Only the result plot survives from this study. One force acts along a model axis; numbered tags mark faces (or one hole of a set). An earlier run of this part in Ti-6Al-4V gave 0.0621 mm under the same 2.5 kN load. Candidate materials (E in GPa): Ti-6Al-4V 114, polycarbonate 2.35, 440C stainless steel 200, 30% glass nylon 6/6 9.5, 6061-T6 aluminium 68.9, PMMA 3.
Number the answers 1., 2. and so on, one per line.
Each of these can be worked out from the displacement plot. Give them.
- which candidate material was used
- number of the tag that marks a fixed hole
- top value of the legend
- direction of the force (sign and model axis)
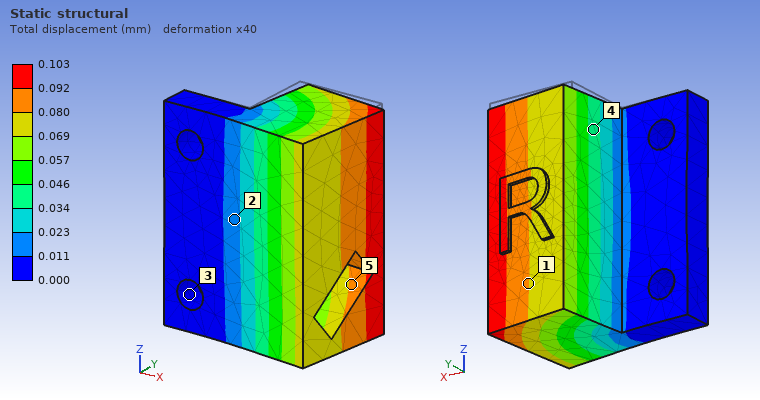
1. 6061-T6 aluminium
2. 3
3. 0.103 mm
4. +X
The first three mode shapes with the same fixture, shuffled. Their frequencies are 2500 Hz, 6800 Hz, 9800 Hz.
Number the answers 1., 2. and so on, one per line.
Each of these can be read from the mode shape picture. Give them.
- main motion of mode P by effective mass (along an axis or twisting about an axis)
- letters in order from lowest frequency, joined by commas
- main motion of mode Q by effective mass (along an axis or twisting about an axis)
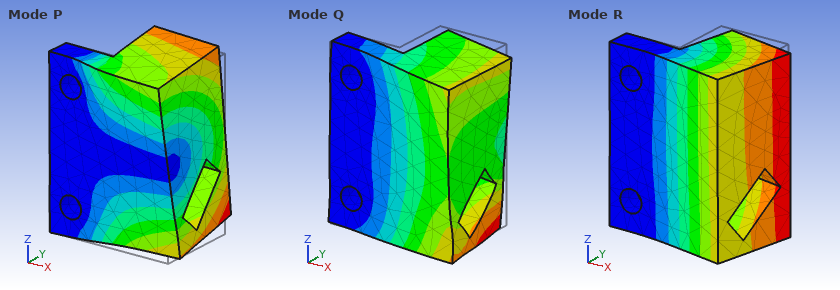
1. along Z
2. R, P, Q
3. along Z
